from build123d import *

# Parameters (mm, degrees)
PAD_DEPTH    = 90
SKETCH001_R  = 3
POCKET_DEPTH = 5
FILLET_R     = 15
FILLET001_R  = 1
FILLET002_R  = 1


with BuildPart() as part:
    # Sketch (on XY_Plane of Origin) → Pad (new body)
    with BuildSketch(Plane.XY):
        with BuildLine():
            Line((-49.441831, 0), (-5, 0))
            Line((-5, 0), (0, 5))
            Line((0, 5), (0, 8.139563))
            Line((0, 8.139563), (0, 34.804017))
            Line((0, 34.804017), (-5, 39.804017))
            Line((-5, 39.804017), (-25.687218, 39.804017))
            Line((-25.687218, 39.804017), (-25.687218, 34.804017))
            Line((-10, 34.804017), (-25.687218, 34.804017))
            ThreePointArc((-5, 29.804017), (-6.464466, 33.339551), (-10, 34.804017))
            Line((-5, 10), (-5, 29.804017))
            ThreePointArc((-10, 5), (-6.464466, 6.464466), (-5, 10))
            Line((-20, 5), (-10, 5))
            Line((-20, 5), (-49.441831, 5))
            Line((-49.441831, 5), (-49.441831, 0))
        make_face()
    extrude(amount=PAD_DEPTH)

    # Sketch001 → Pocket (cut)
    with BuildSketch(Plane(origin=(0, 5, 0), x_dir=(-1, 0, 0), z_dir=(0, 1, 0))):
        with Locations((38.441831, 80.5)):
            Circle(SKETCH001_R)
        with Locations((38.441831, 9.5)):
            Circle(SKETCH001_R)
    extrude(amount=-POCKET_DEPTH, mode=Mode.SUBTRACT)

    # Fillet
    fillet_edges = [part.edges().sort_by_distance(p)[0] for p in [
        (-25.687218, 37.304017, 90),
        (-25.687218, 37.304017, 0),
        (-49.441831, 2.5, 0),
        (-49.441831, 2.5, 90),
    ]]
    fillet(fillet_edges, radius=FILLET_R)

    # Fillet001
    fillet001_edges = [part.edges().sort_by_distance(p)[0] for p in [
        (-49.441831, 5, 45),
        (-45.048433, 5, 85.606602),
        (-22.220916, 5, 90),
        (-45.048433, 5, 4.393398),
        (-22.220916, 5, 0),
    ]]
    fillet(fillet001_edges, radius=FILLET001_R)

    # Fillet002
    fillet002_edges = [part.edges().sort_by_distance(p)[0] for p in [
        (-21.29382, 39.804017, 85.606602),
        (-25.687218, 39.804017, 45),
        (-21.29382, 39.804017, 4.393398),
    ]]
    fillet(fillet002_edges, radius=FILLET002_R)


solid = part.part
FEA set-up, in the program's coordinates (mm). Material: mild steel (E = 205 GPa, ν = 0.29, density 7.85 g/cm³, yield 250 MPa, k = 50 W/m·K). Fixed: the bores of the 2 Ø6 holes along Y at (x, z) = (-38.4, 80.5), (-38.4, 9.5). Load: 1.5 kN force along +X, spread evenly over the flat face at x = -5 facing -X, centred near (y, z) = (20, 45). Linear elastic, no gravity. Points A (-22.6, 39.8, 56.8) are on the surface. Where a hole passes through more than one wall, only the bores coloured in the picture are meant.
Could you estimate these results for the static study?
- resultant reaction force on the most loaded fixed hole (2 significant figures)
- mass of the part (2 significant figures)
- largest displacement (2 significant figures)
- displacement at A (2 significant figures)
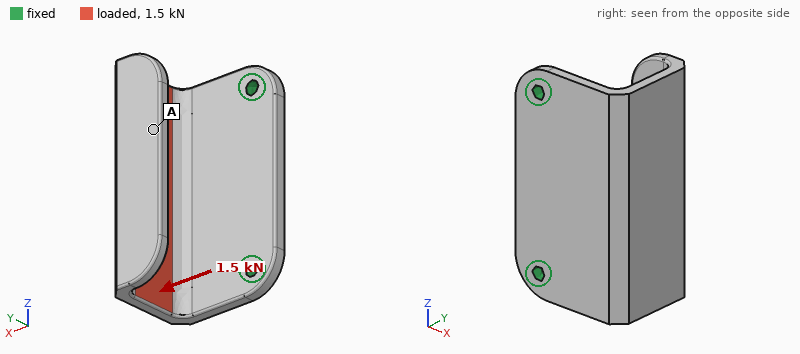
790 N
350 g
0.23 mm
0.21 mm
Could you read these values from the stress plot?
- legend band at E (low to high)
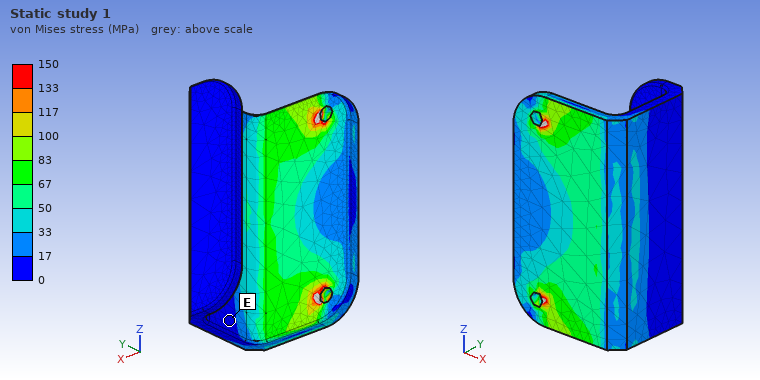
0 to 17 MPa
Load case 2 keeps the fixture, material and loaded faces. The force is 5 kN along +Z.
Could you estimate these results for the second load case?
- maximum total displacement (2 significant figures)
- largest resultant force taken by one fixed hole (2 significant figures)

0.22 mm
3.6 kN
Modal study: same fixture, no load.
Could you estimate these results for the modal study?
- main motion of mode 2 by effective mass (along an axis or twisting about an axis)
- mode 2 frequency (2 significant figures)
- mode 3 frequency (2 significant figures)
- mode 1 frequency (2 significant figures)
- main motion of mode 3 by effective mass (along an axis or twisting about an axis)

along Z
1400 Hz
1800 Hz
750 Hz
along Y
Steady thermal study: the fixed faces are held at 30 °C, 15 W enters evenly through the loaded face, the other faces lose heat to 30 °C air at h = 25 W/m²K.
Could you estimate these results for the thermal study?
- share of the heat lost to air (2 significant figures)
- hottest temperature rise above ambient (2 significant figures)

45 %
24 K
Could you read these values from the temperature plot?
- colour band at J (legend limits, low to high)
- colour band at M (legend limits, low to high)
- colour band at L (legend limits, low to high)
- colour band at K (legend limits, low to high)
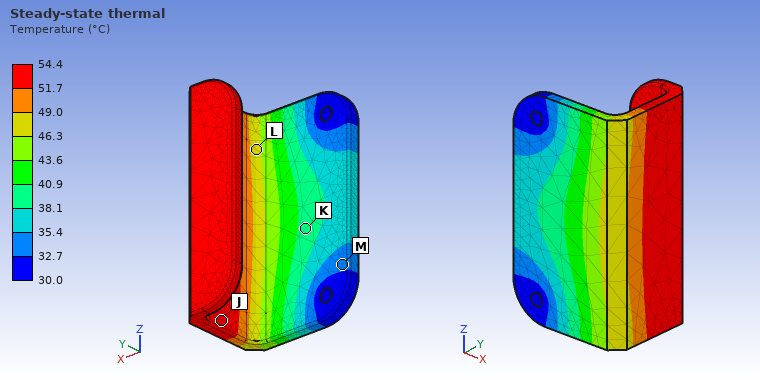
51.7 to 54.4 °C
32.7 to 35.4 °C
46.3 to 49.0 °C
38.1 to 40.9 °C
